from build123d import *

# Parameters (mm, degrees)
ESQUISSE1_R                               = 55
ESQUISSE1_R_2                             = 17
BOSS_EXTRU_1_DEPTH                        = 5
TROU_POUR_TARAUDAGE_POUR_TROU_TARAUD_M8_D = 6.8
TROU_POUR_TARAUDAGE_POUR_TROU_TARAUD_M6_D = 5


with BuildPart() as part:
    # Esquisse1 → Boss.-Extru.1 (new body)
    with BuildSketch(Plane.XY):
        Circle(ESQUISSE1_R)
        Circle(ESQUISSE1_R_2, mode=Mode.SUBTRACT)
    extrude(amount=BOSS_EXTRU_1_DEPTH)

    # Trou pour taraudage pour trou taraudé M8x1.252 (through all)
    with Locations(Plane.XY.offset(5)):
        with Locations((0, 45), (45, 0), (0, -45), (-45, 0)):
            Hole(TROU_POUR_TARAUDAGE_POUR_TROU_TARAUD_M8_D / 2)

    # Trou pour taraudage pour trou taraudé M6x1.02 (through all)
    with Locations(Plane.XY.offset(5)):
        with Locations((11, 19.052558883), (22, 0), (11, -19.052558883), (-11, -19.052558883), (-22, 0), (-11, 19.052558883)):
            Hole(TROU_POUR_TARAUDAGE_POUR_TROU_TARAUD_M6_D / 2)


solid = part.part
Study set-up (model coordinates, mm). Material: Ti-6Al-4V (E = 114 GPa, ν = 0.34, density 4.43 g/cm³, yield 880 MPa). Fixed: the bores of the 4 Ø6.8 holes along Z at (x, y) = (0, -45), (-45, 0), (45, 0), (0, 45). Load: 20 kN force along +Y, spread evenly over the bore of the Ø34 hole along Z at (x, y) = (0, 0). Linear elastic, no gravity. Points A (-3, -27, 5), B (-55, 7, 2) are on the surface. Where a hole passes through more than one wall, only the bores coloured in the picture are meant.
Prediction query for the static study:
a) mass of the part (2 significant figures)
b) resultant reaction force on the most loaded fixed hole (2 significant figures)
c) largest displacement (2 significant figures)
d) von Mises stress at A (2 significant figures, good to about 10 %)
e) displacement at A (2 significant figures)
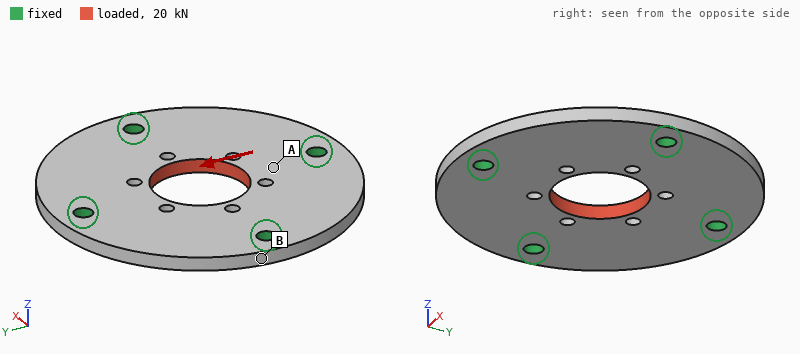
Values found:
180 g
6.0 kN
18 µm
57 MPa
9.0 µm
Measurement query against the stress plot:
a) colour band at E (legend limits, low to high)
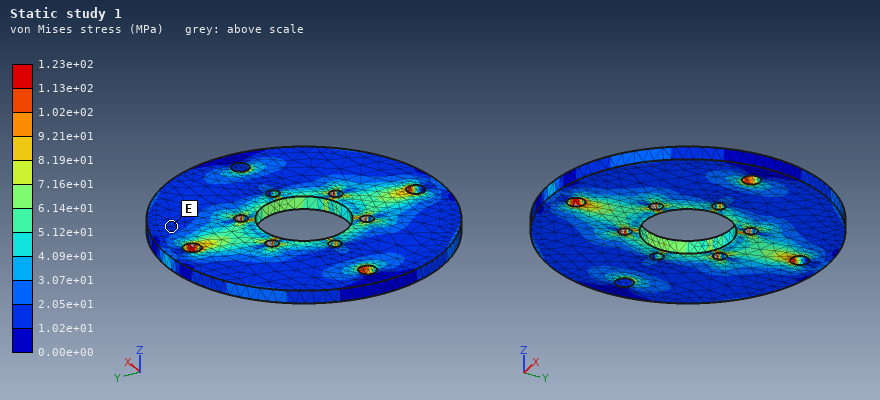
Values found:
1.02e+01 to 2.05e+01 MPa
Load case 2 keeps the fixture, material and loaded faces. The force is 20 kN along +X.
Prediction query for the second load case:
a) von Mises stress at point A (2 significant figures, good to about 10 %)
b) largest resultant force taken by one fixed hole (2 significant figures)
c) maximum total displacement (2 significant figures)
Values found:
13 MPa
6.1 kN
18 µm
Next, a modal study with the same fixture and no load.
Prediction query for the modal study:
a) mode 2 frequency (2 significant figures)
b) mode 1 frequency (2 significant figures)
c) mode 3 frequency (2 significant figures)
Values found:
5300 Hz
5000 Hz
5300 Hz
